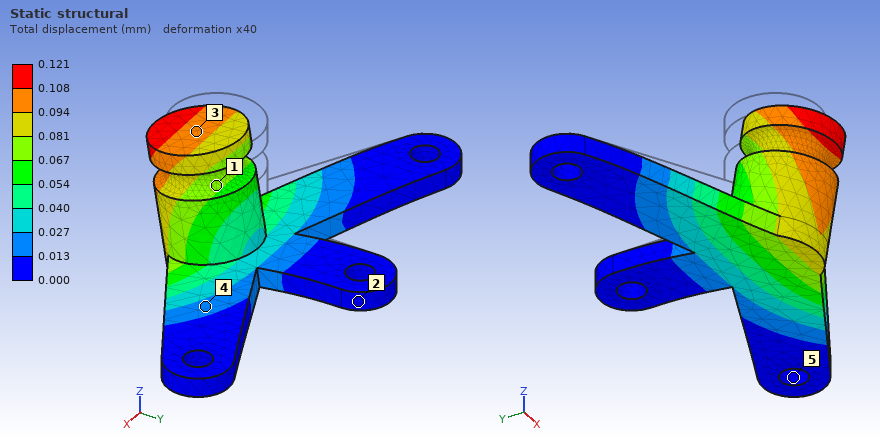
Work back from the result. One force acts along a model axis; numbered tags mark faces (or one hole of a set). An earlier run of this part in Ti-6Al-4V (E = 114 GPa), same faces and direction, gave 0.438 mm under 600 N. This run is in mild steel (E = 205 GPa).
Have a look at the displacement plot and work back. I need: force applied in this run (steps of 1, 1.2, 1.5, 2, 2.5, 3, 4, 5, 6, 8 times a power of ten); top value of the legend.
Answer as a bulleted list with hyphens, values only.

- 300 N
- 0.121 mm
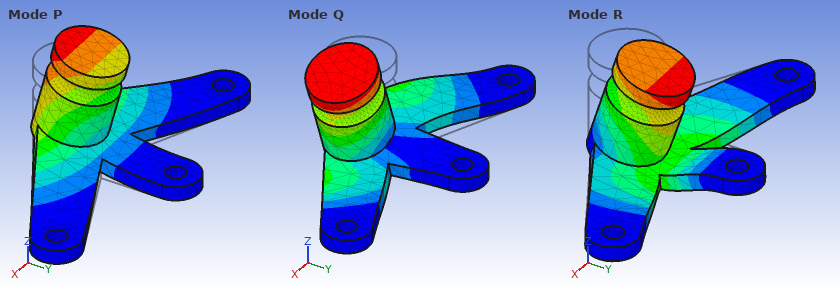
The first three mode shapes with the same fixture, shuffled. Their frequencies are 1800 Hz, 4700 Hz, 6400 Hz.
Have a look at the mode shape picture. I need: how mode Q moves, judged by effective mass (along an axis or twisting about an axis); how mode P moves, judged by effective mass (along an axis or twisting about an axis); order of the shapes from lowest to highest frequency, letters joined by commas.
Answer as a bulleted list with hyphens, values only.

- along X
- along Z
- P, Q, R
